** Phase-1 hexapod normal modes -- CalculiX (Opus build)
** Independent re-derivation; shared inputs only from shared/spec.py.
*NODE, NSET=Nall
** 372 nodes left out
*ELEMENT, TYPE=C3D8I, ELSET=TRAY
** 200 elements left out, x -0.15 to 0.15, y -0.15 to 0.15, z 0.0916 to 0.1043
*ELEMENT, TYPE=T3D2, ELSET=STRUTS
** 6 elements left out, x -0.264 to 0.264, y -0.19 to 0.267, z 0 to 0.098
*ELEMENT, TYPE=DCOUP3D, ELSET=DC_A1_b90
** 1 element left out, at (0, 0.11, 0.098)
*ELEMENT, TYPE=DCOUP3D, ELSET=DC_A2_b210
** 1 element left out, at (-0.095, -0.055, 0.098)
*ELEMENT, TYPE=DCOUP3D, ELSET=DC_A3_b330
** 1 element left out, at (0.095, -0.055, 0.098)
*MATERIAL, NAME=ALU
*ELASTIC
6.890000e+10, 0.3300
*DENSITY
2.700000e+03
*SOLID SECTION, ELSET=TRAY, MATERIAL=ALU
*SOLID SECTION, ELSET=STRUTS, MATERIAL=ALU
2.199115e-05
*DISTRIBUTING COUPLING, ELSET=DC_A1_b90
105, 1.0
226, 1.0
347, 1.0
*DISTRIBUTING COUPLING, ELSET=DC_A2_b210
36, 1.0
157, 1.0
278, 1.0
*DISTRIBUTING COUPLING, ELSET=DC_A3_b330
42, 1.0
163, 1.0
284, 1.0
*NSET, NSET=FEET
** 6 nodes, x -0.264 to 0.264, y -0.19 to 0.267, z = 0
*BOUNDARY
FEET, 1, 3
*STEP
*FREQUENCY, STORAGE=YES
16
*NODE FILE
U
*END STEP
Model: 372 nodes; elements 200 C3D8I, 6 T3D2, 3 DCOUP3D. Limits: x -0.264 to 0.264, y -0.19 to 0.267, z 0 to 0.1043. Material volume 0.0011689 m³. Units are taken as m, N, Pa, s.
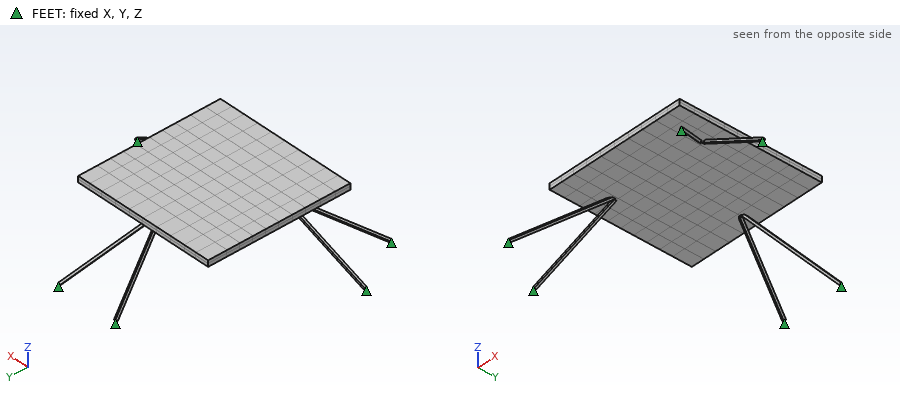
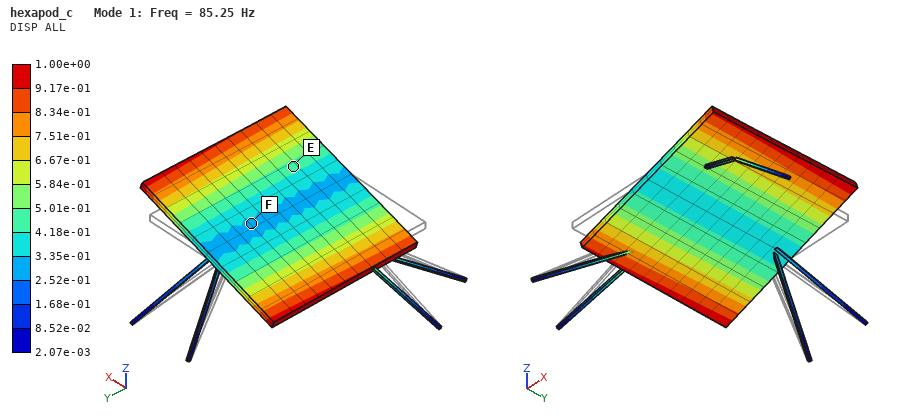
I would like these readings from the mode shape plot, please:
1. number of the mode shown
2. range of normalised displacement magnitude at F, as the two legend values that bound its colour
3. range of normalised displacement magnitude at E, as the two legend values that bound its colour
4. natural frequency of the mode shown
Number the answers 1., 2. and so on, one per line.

1. 1
2. 2.52e-01 to 3.35e-01
3. 4.18e-01 to 5.01e-01
4. 85.25 Hz
